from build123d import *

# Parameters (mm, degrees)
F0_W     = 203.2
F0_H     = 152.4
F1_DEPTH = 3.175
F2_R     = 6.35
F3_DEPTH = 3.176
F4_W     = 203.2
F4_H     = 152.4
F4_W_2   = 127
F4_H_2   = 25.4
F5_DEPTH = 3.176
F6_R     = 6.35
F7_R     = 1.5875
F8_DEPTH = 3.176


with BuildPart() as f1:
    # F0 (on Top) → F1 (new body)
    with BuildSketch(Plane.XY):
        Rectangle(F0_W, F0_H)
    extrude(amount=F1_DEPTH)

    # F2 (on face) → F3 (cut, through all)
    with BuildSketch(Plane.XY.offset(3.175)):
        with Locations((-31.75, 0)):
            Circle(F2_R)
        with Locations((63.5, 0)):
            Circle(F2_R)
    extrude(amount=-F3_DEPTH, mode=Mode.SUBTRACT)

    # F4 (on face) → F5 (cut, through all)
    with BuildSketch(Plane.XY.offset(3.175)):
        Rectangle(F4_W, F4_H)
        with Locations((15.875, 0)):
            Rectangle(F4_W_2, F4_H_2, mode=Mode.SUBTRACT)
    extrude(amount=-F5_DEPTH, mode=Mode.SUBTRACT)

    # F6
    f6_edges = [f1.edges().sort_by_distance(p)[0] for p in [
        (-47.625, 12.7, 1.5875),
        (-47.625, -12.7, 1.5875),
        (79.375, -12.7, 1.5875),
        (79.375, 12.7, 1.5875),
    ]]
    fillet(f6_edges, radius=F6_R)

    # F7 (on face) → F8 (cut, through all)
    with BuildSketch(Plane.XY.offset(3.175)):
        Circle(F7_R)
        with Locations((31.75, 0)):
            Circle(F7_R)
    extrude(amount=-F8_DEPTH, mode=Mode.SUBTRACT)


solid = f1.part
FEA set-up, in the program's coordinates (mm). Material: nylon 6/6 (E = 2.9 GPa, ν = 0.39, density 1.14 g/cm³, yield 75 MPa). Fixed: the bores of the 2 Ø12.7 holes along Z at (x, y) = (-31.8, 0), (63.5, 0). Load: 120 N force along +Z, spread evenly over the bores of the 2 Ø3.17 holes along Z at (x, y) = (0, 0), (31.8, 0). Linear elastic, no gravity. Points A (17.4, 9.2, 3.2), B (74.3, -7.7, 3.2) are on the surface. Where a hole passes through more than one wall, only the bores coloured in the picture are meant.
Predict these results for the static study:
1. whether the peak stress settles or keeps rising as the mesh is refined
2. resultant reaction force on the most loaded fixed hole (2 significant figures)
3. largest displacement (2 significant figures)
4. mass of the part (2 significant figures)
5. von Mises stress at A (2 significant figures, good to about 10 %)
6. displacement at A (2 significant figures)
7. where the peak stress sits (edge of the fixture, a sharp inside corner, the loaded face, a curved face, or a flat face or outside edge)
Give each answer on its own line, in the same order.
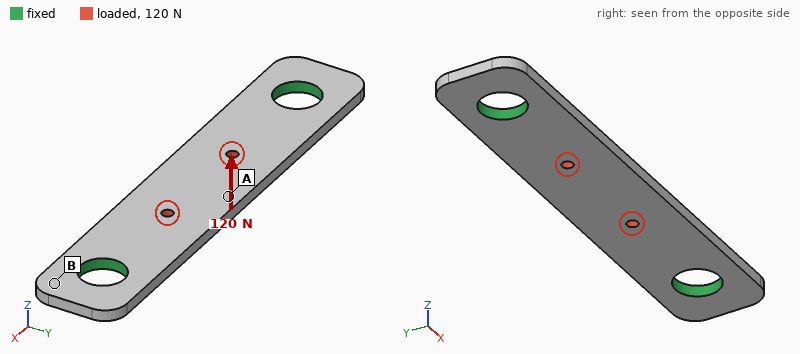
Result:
keeps rising
60 N
1.3 mm
11 g
11 MPa
1.3 mm
edge of the fixture
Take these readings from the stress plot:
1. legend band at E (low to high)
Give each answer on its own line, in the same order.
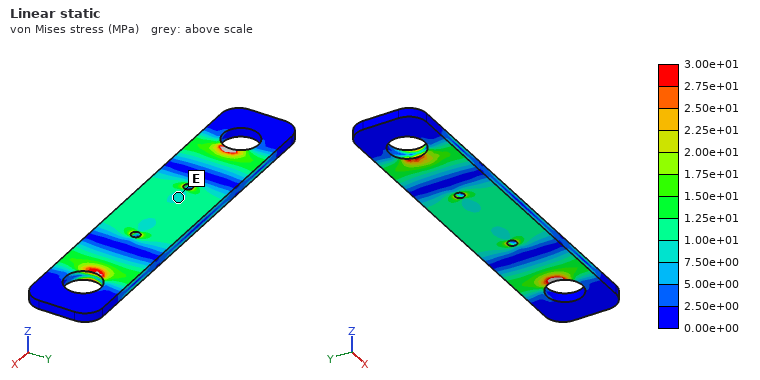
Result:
7.50e+00 to 1.00e+01 MPa
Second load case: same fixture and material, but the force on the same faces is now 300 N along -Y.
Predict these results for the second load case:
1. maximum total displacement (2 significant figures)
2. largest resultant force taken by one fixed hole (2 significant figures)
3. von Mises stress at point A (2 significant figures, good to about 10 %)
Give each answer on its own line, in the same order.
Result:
0.15 mm
150 N
3.6 MPa
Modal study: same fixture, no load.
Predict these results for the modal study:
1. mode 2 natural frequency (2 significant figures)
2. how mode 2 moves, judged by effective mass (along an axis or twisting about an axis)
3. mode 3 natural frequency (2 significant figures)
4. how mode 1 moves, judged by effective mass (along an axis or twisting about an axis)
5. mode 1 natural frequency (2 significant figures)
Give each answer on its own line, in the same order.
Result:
1500 Hz
twisting about X
2000 Hz
along Z
730 Hz
